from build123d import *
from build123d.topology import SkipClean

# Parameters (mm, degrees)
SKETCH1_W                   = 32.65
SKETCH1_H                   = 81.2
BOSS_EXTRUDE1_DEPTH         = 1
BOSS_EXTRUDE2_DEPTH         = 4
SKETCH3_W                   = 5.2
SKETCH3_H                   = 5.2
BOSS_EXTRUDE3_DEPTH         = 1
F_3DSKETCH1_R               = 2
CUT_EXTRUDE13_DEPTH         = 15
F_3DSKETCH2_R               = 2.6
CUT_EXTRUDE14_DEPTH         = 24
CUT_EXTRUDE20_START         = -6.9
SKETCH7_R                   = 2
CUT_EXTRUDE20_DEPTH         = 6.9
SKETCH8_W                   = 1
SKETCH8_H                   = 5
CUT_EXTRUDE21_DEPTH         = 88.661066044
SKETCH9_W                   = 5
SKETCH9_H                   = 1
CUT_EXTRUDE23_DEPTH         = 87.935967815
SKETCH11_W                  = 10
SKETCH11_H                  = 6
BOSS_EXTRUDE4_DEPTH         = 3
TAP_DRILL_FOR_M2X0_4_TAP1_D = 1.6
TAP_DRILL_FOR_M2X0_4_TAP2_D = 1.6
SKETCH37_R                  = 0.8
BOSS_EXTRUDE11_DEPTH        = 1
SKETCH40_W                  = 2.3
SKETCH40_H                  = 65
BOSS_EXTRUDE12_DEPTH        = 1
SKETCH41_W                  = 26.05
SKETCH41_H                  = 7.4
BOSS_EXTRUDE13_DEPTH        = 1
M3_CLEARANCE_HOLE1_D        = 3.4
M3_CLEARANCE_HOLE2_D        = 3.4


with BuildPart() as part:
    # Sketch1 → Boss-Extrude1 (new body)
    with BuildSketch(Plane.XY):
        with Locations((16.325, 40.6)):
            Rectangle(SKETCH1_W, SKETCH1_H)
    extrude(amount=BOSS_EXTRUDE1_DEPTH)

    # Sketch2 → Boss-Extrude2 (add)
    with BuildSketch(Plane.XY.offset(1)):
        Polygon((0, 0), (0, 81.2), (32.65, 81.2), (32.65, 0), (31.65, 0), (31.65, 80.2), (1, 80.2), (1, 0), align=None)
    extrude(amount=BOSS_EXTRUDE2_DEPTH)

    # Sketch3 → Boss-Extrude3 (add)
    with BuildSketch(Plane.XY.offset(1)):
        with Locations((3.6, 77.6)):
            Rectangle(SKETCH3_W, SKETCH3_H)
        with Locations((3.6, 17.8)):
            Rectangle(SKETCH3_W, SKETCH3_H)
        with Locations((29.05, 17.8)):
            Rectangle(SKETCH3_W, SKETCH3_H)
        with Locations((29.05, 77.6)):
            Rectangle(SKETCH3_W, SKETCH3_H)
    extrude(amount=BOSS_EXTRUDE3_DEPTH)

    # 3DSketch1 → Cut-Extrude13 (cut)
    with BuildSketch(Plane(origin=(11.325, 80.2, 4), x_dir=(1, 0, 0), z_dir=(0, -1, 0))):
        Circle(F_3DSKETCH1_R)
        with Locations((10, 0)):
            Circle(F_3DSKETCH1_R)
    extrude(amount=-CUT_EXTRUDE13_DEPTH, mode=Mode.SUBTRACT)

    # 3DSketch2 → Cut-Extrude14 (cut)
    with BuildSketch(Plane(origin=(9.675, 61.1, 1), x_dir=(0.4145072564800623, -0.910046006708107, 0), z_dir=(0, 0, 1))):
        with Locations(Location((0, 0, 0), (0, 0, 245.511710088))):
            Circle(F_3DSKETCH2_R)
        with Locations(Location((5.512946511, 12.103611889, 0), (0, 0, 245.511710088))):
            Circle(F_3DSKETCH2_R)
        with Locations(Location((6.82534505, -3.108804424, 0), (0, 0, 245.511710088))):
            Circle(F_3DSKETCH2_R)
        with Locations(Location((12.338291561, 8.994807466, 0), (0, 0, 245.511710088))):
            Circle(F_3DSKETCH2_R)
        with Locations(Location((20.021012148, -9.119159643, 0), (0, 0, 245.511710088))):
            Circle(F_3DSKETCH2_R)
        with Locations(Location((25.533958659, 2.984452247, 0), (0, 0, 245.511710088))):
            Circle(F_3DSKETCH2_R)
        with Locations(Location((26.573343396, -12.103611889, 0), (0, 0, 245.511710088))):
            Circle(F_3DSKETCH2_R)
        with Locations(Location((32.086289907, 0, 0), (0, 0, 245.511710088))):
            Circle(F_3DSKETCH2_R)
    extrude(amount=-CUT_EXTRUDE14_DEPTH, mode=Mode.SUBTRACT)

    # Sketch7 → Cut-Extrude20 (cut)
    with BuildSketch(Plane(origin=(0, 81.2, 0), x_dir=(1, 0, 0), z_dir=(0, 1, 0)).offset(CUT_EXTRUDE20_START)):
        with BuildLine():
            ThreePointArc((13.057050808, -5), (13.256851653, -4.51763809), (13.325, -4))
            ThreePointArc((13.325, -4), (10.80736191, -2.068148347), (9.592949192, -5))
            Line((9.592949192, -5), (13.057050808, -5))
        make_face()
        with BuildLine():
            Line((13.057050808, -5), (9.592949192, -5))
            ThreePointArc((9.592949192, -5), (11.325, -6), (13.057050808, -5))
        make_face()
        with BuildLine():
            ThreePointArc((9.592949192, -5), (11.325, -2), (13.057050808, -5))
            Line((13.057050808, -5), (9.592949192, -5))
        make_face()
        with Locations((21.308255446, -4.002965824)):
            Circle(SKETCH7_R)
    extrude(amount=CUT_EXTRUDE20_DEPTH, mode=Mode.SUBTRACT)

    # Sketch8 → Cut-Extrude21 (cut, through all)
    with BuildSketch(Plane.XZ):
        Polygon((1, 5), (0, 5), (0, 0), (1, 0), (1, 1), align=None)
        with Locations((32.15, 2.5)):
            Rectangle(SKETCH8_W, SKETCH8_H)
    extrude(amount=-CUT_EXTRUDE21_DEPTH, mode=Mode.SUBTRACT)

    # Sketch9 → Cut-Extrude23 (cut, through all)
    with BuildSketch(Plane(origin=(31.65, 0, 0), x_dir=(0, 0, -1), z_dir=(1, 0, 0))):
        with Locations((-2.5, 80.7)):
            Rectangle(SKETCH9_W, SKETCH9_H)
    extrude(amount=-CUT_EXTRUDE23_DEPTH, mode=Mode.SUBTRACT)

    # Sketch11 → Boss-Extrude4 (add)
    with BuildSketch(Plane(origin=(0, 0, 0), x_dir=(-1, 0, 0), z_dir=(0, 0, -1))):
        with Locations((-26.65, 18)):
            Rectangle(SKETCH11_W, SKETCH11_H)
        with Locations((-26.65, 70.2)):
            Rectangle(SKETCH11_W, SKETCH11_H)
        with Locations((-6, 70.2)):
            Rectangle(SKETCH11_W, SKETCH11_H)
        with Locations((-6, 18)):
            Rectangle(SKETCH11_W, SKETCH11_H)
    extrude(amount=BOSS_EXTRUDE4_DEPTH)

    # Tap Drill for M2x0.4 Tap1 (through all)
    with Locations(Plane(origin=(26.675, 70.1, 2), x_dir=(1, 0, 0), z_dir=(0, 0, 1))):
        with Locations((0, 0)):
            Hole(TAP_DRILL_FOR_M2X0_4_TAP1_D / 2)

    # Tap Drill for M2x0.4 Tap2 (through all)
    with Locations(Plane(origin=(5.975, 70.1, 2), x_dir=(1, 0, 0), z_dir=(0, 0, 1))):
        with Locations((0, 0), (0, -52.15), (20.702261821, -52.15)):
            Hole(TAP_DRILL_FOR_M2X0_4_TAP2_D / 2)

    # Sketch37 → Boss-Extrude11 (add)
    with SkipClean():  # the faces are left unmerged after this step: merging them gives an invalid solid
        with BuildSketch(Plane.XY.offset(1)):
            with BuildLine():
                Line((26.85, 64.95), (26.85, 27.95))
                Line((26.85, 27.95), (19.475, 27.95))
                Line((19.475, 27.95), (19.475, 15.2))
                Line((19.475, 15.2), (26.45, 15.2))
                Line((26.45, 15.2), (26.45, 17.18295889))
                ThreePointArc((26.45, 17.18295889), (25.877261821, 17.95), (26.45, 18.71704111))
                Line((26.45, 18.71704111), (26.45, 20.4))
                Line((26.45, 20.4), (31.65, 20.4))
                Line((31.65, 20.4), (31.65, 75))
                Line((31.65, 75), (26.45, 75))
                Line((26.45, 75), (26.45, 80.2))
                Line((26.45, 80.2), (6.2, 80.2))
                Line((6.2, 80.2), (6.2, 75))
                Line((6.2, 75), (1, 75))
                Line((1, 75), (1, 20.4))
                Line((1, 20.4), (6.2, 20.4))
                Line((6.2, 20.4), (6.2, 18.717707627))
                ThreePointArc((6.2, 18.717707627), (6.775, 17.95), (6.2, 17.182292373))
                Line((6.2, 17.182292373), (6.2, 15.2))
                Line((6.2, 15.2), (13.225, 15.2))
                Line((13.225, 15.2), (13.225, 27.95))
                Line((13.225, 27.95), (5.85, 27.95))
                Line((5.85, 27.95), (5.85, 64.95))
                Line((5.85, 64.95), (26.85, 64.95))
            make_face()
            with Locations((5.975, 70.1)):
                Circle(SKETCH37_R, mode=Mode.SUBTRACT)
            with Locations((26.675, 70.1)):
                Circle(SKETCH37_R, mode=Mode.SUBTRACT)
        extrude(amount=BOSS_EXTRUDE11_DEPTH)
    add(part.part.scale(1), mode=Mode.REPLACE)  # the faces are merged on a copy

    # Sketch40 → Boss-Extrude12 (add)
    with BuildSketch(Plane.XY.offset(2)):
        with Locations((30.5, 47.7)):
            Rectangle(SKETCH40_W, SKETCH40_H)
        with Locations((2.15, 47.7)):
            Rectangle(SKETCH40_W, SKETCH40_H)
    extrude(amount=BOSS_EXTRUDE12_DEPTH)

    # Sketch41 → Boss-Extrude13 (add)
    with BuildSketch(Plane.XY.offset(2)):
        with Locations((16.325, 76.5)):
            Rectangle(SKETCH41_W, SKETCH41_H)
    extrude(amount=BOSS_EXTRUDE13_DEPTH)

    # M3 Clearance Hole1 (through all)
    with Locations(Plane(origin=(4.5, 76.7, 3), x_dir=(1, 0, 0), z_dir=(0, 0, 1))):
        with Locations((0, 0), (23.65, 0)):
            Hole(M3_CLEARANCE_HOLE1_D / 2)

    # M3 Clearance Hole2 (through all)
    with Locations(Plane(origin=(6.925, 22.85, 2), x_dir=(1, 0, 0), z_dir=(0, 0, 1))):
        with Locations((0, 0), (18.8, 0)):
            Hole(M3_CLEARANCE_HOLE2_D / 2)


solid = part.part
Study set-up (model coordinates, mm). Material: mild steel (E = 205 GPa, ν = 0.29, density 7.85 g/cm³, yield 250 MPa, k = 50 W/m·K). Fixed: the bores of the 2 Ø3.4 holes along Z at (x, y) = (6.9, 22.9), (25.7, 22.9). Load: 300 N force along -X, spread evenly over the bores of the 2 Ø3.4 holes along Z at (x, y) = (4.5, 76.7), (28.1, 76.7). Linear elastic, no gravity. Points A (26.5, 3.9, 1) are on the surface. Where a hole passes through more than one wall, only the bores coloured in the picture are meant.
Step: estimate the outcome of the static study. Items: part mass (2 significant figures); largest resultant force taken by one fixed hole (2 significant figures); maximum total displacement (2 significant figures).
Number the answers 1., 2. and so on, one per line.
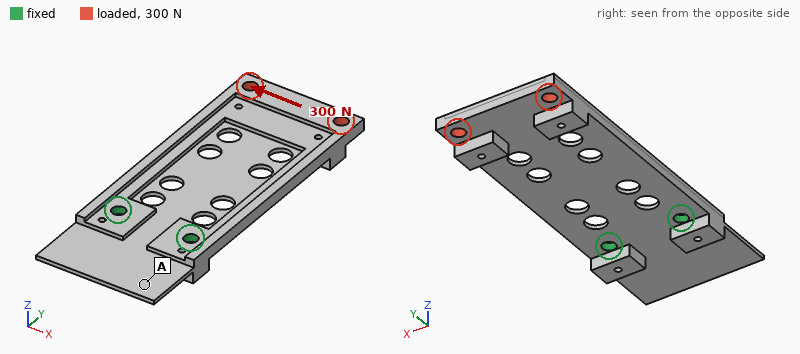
1. 35 g
2. 770 N
3. 74 µm
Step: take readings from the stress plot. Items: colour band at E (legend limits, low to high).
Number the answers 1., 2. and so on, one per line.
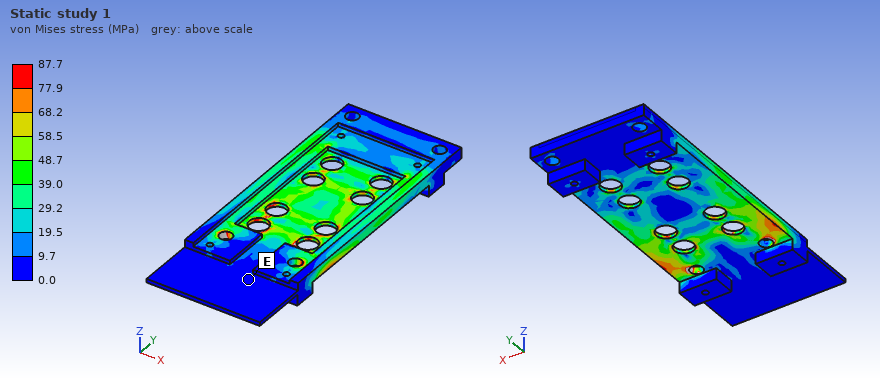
1. 0.0 to 9.7 MPa
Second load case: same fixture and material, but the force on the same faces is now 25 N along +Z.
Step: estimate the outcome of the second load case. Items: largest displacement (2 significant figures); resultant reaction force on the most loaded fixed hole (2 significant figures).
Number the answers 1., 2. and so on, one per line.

1. 0.32 mm
2. 21 N
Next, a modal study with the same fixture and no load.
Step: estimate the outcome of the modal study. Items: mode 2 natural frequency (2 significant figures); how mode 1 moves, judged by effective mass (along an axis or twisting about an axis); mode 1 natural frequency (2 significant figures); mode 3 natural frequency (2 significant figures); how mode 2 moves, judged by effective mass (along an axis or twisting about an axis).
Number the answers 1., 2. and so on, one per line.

1. 1400 Hz
2. along Z
3. 450 Hz
4. 3200 Hz
5. twisting about Y
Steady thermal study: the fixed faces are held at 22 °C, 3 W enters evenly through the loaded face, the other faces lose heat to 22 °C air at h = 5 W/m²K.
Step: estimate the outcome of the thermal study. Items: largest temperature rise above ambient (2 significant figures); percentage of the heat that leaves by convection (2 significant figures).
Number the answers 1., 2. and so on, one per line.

1. 64 K
2. 25 %
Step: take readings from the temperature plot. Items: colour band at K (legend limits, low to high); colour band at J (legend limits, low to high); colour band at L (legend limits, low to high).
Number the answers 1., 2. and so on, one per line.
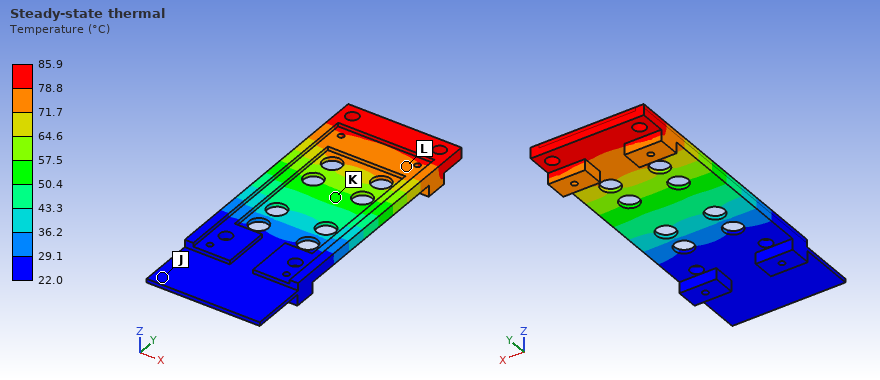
1. 50.4 to 57.5 °C
2. 22.0 to 29.1 °C
3. 71.7 to 78.8 °C
